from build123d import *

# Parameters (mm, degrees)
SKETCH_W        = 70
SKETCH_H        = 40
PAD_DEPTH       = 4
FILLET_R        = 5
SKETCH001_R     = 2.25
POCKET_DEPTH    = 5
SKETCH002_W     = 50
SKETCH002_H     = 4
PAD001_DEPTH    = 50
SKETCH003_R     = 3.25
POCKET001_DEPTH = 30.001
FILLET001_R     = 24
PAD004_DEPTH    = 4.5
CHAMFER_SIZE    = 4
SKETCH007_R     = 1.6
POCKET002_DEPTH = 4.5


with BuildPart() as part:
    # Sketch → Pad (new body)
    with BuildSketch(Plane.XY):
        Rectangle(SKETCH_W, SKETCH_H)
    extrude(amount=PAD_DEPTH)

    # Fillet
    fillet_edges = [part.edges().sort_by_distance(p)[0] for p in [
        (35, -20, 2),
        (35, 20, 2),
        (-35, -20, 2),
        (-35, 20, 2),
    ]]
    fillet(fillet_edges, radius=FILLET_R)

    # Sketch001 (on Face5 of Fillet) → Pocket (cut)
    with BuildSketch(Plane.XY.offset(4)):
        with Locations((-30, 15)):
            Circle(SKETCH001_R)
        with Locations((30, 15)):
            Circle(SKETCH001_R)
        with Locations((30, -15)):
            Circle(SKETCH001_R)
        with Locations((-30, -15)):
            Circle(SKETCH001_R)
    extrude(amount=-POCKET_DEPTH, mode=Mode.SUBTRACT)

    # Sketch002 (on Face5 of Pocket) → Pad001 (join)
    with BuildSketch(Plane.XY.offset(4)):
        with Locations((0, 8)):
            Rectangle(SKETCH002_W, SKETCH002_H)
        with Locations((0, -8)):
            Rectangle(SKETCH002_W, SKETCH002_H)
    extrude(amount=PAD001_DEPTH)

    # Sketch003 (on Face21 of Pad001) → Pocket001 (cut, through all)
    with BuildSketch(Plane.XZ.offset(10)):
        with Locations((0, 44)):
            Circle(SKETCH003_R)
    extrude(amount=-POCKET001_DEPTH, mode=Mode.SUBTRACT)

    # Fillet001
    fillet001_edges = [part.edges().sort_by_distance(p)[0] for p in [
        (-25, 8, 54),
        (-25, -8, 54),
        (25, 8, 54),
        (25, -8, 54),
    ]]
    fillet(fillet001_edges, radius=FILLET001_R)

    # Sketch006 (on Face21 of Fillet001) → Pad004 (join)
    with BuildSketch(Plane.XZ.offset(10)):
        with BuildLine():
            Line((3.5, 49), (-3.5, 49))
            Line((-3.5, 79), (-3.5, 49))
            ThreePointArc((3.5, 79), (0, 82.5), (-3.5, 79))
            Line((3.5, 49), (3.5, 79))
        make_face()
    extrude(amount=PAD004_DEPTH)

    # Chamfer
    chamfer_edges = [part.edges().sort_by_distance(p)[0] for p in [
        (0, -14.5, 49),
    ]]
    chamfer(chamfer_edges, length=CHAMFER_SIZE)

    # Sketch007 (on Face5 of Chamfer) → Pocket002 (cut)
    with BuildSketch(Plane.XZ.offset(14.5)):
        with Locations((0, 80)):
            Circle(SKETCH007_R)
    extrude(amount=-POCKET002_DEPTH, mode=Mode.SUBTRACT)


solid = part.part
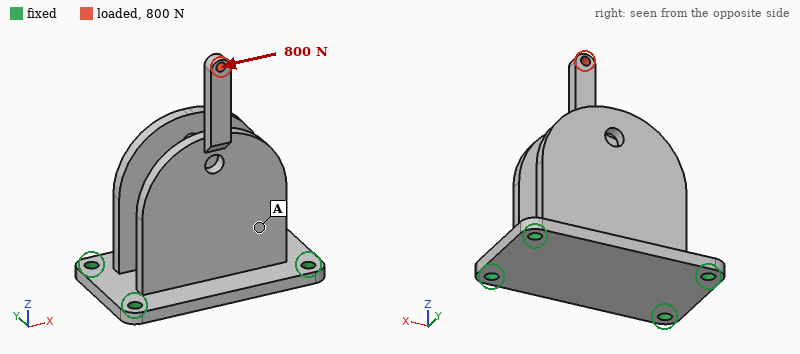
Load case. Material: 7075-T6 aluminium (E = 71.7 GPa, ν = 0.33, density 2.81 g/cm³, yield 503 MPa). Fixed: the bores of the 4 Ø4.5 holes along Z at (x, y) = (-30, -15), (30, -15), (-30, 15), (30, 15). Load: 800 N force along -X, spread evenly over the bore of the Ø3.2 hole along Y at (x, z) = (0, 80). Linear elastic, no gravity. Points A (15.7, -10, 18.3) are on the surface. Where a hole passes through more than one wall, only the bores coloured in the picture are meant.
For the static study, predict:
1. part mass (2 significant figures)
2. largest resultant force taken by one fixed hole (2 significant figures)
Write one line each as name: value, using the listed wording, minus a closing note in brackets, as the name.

part mass: 83 g
largest resultant force taken by one fixed hole: 990 N
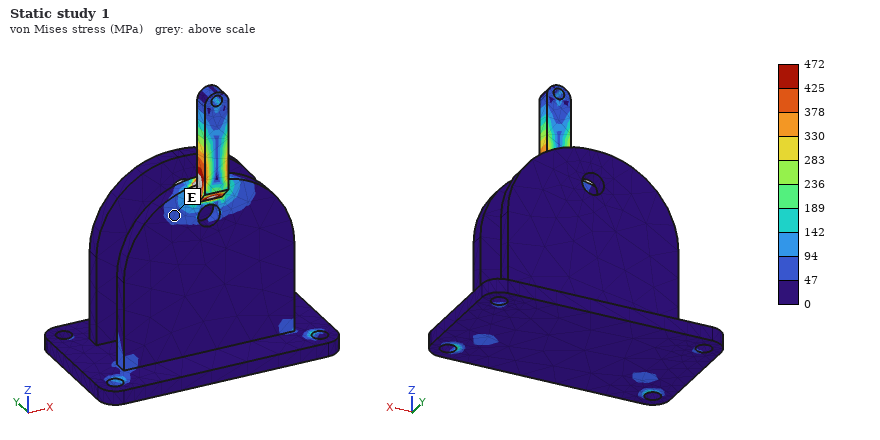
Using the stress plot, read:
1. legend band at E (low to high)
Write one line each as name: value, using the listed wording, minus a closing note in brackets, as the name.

legend band at E: 47 to 94 MPa
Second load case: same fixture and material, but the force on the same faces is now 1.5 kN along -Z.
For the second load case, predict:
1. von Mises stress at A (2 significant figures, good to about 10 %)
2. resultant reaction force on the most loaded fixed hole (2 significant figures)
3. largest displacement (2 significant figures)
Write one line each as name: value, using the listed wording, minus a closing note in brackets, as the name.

von Mises stress at A: 55 MPa
resultant reaction force on the most loaded fixed hole: 760 N
largest displacement: 1.3 mm
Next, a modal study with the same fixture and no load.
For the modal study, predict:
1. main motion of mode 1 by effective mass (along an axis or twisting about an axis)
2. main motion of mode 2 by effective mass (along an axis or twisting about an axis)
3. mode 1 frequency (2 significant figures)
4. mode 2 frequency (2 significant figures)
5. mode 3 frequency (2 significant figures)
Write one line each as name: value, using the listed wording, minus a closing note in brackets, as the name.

main motion of mode 1 by effective mass: along Y
main motion of mode 2 by effective mass: along Y
mode 1 frequency: 960 Hz
mode 2 frequency: 1400 Hz
mode 3 frequency: 3200 Hz
